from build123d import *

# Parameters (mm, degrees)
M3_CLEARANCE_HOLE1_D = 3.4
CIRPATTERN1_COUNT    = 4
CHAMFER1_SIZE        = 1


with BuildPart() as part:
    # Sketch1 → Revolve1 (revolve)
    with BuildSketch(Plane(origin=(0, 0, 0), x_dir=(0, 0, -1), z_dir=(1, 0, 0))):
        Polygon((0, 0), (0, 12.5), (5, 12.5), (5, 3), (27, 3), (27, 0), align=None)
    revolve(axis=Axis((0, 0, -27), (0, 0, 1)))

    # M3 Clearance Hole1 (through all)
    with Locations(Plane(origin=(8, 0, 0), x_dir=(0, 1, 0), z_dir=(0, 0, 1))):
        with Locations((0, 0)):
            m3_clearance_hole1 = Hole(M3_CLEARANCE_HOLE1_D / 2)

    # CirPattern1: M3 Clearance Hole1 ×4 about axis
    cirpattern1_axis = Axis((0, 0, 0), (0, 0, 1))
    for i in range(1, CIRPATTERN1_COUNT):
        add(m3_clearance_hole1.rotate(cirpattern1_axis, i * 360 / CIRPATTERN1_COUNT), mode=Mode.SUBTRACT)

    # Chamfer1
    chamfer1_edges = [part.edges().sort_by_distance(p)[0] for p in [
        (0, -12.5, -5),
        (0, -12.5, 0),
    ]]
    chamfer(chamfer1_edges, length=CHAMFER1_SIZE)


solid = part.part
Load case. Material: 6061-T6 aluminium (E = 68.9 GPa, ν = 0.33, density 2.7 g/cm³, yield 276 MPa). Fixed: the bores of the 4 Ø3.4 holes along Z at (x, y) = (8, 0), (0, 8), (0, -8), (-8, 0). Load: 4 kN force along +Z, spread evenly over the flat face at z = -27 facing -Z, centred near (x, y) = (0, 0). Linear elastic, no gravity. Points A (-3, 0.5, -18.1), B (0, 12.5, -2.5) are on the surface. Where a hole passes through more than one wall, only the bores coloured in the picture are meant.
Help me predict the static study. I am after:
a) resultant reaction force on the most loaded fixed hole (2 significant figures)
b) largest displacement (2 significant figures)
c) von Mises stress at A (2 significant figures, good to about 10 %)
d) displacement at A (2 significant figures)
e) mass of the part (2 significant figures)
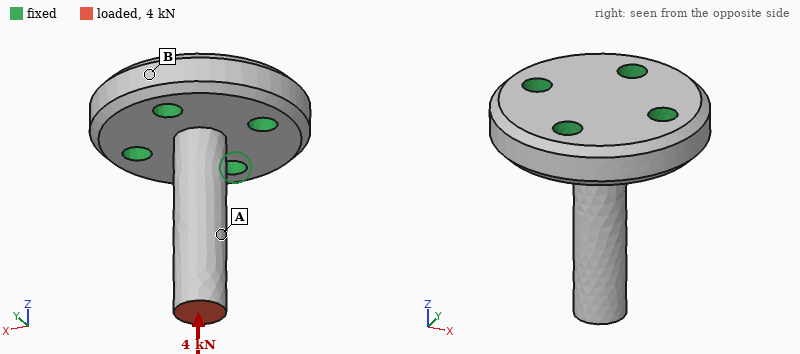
1.0 kN
55 µm
140 MPa
37 µm
7.6 g
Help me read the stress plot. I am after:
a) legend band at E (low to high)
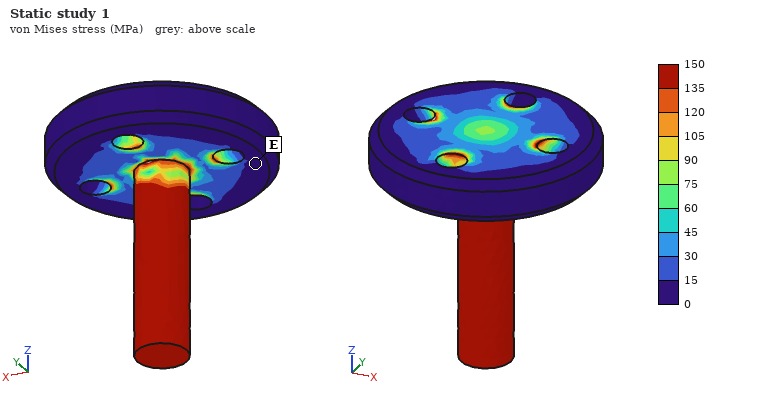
0 to 15 MPa
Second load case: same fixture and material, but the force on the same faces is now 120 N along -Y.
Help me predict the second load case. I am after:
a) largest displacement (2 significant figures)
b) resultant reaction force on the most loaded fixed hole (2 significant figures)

0.12 mm
210 N
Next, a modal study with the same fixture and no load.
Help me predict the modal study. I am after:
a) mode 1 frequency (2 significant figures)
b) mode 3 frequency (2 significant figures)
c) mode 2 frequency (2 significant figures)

7500 Hz
34 kHz
7500 Hz
